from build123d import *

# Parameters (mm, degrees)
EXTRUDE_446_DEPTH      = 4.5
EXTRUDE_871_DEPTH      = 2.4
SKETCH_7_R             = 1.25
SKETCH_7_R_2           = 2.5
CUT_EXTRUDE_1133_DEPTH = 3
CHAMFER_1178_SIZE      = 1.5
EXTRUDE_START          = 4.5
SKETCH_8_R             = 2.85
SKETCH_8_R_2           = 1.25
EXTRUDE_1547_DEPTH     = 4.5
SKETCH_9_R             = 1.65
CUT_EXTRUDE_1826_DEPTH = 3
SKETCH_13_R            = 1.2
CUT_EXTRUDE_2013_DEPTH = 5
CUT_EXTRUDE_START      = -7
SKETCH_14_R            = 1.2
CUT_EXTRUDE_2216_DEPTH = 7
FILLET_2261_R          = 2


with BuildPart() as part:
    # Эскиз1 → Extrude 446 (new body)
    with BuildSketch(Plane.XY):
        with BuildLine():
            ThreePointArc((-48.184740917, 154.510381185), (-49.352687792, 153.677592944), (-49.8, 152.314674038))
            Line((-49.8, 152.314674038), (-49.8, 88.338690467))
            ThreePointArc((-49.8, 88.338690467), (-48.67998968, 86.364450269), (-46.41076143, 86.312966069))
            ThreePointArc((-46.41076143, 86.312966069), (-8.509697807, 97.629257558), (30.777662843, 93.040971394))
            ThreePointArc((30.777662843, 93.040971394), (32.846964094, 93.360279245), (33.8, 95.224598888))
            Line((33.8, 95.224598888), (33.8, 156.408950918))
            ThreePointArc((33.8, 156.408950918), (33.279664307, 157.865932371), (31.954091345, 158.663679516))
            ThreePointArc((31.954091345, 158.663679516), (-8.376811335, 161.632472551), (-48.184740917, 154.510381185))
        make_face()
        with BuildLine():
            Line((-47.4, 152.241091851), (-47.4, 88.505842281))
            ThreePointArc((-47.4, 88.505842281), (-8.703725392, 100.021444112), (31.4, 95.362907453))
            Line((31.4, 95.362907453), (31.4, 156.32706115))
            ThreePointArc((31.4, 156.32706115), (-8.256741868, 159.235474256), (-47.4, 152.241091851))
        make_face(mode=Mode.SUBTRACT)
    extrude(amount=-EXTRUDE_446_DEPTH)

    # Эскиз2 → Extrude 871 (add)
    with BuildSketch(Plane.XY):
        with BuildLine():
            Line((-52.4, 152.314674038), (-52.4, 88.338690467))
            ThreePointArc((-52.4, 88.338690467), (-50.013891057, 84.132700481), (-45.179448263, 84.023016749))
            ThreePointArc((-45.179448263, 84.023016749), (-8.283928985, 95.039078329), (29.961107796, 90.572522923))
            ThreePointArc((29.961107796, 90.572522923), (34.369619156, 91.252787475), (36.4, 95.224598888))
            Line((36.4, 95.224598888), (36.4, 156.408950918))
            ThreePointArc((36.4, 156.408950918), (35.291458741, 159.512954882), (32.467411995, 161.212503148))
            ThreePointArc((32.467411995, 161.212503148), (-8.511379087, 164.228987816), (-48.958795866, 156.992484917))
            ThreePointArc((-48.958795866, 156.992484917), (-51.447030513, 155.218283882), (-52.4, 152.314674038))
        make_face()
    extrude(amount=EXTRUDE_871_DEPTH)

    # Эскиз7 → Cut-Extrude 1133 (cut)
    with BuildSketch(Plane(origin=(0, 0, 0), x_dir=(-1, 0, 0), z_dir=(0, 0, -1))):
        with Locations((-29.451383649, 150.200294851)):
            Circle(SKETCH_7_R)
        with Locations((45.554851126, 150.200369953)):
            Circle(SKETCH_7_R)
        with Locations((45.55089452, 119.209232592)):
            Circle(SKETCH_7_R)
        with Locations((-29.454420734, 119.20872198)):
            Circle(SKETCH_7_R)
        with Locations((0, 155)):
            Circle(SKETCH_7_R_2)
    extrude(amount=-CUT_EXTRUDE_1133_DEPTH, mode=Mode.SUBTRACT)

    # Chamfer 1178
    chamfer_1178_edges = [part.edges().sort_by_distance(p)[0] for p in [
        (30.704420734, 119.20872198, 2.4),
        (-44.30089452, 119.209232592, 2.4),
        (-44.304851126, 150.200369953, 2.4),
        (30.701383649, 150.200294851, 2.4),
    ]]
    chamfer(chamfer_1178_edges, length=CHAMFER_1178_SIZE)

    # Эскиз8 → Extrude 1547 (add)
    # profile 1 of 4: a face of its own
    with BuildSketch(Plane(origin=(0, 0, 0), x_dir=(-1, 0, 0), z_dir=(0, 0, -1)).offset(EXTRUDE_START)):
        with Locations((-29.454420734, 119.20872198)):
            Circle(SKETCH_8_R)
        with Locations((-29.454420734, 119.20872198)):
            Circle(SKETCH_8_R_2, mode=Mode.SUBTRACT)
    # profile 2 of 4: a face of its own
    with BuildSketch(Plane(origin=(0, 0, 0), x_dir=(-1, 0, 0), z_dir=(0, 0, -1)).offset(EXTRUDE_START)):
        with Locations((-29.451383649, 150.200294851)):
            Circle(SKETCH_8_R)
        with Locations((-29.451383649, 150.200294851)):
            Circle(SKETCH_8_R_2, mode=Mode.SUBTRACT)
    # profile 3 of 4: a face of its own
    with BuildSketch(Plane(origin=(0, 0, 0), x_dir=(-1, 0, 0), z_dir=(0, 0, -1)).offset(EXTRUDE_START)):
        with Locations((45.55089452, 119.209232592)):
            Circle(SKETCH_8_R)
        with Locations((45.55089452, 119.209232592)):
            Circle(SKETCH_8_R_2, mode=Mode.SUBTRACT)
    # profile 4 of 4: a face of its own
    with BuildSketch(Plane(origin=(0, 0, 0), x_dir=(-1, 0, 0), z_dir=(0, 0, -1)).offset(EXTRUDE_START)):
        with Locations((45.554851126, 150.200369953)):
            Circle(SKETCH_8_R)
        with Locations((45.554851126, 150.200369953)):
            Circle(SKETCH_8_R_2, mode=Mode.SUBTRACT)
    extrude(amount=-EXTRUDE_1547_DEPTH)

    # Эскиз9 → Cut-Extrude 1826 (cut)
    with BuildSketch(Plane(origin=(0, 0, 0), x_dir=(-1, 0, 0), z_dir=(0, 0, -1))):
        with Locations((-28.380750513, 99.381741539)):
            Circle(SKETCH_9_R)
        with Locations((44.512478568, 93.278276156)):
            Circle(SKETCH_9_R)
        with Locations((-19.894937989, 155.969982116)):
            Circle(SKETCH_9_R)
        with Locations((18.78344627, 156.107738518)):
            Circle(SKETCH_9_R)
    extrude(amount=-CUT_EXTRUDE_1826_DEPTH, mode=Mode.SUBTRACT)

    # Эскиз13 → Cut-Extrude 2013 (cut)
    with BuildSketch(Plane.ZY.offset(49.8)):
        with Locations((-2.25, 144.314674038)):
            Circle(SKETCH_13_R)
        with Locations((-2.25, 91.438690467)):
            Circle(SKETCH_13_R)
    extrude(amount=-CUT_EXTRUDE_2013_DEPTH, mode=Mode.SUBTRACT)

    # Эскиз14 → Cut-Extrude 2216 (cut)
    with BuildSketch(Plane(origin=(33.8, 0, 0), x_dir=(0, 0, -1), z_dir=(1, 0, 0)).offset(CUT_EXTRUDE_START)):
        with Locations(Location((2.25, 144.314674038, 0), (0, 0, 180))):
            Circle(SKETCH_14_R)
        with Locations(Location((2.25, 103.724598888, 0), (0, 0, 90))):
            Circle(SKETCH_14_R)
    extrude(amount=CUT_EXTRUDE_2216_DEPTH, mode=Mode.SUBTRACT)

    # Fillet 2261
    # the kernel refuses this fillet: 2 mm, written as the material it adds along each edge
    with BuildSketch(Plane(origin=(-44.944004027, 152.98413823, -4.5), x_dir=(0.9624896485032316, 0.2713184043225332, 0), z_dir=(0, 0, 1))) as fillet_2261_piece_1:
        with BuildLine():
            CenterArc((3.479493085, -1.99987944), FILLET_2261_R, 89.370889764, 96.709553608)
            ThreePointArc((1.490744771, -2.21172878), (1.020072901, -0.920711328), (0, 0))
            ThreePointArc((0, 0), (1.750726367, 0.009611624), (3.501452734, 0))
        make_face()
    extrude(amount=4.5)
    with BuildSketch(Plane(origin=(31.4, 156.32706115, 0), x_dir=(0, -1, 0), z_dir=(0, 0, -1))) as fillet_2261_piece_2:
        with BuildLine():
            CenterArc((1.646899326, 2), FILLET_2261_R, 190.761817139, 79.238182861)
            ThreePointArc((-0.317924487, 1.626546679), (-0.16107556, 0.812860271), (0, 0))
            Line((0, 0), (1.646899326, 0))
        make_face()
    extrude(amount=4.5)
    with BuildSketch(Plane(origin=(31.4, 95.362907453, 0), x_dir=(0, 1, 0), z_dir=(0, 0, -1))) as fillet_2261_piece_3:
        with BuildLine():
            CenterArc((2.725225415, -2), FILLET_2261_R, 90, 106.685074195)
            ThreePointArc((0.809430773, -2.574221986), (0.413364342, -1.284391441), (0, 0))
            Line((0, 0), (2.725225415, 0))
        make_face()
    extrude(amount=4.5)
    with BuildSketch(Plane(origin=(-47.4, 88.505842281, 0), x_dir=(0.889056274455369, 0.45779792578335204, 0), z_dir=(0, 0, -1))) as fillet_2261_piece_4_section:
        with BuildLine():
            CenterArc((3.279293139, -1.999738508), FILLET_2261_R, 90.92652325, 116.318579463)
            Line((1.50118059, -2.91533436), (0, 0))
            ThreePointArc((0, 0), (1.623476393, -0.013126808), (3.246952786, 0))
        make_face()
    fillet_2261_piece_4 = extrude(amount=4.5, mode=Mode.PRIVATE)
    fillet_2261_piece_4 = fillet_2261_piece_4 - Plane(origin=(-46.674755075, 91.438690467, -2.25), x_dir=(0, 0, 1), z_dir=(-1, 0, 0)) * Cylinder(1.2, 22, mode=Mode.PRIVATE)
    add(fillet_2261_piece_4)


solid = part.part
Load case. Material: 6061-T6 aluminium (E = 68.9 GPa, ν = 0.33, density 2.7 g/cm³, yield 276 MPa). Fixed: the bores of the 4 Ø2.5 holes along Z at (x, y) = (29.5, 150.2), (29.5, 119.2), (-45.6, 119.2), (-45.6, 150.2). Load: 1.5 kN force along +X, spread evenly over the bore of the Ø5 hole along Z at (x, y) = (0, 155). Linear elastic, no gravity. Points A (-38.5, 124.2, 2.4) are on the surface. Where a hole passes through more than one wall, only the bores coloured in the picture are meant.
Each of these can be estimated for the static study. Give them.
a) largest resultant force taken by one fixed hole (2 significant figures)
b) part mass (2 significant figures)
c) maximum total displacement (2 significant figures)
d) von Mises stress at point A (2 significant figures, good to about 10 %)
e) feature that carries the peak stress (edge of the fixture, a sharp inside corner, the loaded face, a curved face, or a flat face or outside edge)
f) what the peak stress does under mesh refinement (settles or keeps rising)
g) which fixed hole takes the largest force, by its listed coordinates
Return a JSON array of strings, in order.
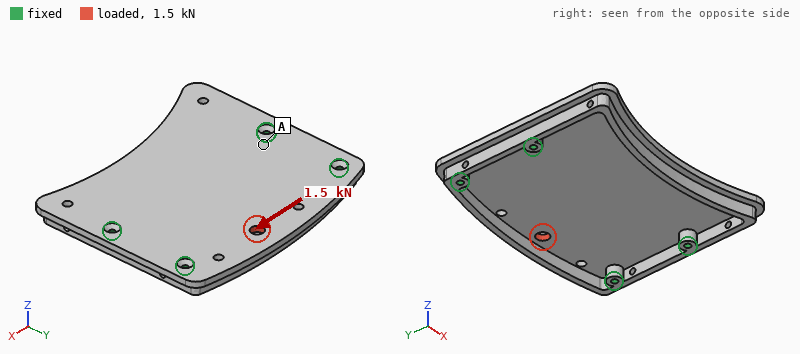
["650 N", "49 g", "11 µm", "5.4 MPa", "edge of the fixture", "keeps rising", "(29.5, 150.2)"]
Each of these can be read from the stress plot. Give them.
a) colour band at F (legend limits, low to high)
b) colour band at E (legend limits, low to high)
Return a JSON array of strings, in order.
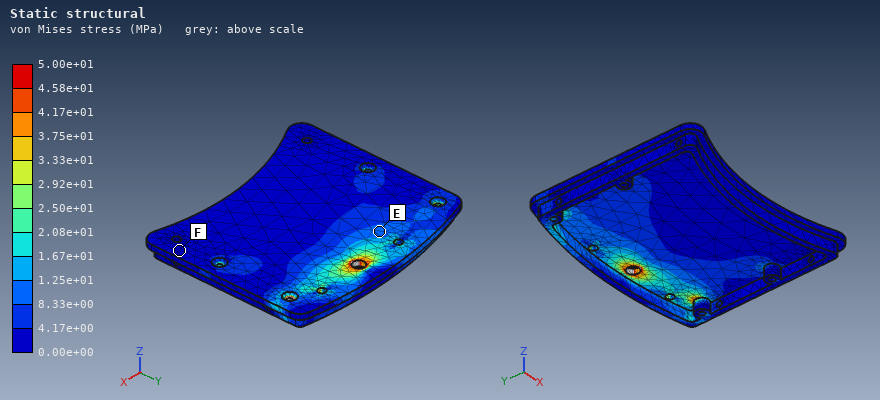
["0.00e+00 to 4.17e+00 MPa", "8.33e+00 to 1.25e+01 MPa"]
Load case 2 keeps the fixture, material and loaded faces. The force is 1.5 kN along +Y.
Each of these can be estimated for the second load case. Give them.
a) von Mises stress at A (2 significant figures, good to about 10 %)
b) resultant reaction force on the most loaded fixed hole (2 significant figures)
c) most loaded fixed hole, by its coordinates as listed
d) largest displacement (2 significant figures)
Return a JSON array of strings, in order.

["11 MPa", "520 N", "(29.5, 119.2)", "20 µm"]
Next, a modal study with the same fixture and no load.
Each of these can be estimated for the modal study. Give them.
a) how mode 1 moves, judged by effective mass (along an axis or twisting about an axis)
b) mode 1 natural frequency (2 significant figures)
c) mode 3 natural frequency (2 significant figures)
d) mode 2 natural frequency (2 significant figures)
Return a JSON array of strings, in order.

["along Z", "2000 Hz", "3700 Hz", "3000 Hz"]
